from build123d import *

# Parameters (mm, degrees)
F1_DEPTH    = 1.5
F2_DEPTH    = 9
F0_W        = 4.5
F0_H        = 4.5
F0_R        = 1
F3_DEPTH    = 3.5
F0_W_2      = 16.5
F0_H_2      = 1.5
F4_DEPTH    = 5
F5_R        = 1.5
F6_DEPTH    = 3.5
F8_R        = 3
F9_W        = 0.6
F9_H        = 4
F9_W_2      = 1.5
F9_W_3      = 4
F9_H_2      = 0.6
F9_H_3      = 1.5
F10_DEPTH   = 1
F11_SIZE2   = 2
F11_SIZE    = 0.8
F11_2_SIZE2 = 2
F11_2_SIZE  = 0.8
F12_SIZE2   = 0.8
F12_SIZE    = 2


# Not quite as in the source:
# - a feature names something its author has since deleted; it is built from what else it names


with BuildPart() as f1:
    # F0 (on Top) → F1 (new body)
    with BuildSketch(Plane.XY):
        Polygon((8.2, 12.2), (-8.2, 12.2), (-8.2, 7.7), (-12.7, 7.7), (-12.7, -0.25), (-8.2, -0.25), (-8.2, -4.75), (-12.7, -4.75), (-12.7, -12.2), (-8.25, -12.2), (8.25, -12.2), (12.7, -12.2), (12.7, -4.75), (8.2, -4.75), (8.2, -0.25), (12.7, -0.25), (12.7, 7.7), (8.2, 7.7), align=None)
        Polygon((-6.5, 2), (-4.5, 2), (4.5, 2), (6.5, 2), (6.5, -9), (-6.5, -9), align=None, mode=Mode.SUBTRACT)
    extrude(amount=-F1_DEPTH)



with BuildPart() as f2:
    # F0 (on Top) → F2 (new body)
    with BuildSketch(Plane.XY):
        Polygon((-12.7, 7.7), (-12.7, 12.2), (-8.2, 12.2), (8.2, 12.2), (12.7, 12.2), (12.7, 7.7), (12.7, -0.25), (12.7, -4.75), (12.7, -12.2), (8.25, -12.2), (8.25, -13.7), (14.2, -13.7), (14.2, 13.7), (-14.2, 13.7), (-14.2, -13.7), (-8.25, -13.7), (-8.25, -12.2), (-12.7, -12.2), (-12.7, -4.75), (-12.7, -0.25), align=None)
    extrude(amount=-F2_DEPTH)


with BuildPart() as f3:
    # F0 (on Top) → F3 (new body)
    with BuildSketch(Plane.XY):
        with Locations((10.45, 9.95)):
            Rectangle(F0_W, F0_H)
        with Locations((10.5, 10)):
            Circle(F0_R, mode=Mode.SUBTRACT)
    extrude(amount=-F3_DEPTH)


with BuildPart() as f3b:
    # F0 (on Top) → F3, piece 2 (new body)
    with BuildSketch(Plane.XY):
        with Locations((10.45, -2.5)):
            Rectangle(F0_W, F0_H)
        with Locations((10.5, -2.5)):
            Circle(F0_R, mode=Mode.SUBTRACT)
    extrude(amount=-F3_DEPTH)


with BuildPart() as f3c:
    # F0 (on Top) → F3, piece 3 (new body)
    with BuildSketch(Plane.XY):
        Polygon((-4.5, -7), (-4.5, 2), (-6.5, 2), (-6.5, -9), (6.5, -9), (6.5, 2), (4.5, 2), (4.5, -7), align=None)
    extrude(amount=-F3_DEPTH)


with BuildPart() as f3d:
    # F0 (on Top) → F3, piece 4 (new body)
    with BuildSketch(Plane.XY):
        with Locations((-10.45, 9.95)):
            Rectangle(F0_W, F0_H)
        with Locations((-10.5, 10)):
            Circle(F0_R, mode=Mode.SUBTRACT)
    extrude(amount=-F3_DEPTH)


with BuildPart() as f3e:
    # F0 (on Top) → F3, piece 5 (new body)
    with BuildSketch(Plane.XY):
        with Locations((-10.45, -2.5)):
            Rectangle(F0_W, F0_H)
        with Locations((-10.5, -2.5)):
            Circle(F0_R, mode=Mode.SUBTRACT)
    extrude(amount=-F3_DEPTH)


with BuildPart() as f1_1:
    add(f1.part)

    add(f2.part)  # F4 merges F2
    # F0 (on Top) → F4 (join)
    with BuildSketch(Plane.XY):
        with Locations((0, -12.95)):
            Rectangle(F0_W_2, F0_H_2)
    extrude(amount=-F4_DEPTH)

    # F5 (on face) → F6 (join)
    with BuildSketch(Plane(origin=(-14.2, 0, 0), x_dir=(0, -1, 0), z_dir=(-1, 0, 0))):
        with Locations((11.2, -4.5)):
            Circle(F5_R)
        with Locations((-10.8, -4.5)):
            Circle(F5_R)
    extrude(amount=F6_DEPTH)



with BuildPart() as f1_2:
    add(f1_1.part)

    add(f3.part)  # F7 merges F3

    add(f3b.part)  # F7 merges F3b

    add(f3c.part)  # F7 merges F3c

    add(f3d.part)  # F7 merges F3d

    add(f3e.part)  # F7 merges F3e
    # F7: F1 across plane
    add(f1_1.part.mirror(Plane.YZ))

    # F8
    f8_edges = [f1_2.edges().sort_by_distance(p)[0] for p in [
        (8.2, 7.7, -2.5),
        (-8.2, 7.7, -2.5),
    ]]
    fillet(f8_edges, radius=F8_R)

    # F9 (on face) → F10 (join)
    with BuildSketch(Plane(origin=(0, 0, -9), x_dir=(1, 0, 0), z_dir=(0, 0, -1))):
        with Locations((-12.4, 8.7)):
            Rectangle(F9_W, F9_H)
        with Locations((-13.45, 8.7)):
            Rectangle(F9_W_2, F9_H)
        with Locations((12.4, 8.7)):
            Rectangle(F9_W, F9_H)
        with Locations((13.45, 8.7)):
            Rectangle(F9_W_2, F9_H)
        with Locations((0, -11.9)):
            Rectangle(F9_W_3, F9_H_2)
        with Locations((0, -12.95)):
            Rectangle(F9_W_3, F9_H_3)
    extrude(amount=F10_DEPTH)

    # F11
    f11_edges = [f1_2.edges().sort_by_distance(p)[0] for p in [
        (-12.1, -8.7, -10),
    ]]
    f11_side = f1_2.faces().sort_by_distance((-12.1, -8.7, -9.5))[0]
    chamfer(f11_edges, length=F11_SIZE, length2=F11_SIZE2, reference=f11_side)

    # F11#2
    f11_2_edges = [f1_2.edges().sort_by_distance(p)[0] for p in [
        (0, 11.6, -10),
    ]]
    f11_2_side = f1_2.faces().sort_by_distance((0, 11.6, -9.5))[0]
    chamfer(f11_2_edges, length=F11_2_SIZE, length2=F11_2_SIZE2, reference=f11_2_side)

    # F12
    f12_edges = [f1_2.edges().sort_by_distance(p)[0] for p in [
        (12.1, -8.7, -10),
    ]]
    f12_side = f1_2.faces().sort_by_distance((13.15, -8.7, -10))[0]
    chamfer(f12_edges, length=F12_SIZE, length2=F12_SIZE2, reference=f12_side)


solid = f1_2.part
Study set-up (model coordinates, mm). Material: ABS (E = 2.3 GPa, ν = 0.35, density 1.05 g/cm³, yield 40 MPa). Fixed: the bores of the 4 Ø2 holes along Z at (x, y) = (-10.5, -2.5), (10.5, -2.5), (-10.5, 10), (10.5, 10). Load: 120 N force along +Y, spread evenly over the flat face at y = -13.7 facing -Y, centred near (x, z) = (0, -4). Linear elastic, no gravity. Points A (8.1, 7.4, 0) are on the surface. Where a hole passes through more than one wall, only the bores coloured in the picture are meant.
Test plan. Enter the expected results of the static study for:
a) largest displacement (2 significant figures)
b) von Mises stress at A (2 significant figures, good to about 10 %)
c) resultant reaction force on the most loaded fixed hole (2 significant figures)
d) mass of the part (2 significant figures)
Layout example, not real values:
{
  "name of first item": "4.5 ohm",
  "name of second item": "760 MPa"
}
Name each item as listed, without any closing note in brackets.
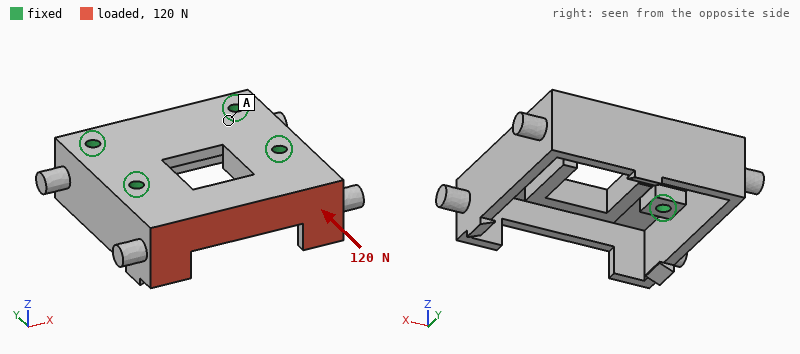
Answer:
{
  "largest displacement": "0.17 mm",
  "von Mises stress at A": "1.0 MPa",
  "resultant reaction force on the most loaded fixed hole": "45 N",
  "mass of the part": "2.6 g"
}
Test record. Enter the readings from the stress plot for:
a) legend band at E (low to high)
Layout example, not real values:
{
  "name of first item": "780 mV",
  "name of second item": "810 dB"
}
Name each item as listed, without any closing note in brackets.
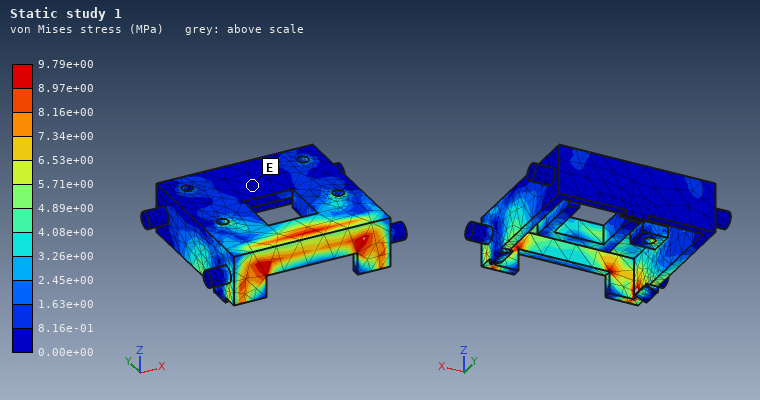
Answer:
{
  "legend band at E": "0.00e+00 to 8.16e-01 MPa"
}
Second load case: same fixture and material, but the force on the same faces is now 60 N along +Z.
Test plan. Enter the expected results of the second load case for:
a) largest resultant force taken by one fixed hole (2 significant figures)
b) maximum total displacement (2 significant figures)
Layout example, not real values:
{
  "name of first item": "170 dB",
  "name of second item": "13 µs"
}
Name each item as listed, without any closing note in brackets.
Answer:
{
  "largest resultant force taken by one fixed hole": "49 N",
  "maximum total displacement": "0.26 mm"
}
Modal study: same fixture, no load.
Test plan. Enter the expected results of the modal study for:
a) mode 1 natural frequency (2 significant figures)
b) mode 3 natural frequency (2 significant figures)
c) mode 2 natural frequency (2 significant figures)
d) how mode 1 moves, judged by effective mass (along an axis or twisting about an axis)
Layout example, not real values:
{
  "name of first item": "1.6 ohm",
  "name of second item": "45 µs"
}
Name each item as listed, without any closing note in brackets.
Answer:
{
  "mode 1 natural frequency": "4200 Hz",
  "mode 3 natural frequency": "5600 Hz",
  "mode 2 natural frequency": "5500 Hz",
  "how mode 1 moves, judged by effective mass": "along Z"
}
